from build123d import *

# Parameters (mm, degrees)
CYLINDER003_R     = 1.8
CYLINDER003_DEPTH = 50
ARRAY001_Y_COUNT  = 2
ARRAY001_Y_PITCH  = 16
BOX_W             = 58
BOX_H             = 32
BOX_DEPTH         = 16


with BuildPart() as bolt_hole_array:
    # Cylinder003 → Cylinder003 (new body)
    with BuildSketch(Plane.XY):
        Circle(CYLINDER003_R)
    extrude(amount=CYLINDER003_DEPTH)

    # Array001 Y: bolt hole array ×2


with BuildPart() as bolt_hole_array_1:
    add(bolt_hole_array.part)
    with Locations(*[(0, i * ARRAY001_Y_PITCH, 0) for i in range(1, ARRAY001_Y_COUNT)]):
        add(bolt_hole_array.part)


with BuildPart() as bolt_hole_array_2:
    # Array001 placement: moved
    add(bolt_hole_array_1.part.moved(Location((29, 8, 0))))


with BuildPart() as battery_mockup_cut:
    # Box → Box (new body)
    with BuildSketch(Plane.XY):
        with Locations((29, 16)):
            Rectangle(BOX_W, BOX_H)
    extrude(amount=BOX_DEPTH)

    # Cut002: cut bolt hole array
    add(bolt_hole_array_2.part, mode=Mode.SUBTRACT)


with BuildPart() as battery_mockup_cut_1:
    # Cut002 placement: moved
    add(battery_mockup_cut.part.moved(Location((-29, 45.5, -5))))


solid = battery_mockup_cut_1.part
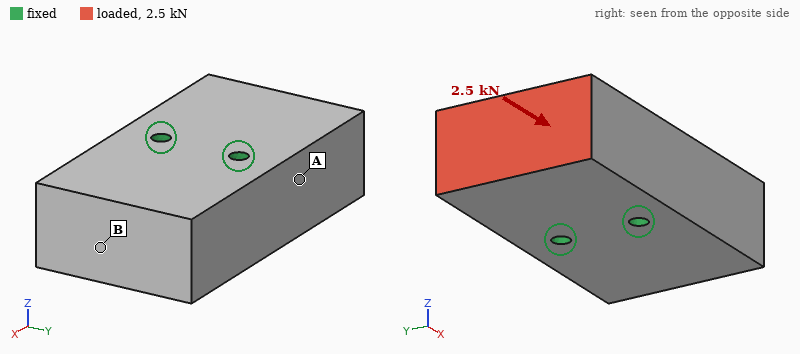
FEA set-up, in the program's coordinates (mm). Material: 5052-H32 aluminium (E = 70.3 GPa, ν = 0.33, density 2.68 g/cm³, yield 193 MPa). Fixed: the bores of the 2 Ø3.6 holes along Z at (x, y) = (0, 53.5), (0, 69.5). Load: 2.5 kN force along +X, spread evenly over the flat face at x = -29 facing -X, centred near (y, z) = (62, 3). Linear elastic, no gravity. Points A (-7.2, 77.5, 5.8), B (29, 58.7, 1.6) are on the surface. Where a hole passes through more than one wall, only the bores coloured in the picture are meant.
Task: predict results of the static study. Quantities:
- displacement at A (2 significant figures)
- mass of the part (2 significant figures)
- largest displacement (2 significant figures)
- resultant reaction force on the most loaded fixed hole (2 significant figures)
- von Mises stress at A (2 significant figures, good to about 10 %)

0.86 µm
79 g
2.2 µm
1.3 kN
3.4 MPa
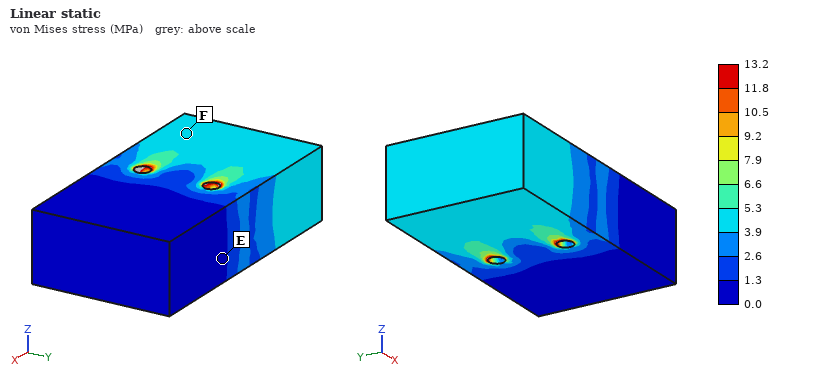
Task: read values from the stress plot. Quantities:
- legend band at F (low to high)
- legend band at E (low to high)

3.9 to 5.3 MPa
0.0 to 1.3 MPa
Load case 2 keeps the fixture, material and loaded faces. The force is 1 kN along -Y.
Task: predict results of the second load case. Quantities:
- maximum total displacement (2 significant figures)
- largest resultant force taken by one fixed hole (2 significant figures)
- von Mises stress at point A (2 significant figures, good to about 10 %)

7.6 µm
1.7 kN
6.2 MPa
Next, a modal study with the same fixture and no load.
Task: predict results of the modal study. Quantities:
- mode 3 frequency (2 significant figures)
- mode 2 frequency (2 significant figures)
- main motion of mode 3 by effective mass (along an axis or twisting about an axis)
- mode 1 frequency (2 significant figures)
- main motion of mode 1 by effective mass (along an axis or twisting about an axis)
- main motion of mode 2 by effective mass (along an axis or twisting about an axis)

15 kHz
14 kHz
twisting about Z
11 kHz
twisting about Y
along Z
